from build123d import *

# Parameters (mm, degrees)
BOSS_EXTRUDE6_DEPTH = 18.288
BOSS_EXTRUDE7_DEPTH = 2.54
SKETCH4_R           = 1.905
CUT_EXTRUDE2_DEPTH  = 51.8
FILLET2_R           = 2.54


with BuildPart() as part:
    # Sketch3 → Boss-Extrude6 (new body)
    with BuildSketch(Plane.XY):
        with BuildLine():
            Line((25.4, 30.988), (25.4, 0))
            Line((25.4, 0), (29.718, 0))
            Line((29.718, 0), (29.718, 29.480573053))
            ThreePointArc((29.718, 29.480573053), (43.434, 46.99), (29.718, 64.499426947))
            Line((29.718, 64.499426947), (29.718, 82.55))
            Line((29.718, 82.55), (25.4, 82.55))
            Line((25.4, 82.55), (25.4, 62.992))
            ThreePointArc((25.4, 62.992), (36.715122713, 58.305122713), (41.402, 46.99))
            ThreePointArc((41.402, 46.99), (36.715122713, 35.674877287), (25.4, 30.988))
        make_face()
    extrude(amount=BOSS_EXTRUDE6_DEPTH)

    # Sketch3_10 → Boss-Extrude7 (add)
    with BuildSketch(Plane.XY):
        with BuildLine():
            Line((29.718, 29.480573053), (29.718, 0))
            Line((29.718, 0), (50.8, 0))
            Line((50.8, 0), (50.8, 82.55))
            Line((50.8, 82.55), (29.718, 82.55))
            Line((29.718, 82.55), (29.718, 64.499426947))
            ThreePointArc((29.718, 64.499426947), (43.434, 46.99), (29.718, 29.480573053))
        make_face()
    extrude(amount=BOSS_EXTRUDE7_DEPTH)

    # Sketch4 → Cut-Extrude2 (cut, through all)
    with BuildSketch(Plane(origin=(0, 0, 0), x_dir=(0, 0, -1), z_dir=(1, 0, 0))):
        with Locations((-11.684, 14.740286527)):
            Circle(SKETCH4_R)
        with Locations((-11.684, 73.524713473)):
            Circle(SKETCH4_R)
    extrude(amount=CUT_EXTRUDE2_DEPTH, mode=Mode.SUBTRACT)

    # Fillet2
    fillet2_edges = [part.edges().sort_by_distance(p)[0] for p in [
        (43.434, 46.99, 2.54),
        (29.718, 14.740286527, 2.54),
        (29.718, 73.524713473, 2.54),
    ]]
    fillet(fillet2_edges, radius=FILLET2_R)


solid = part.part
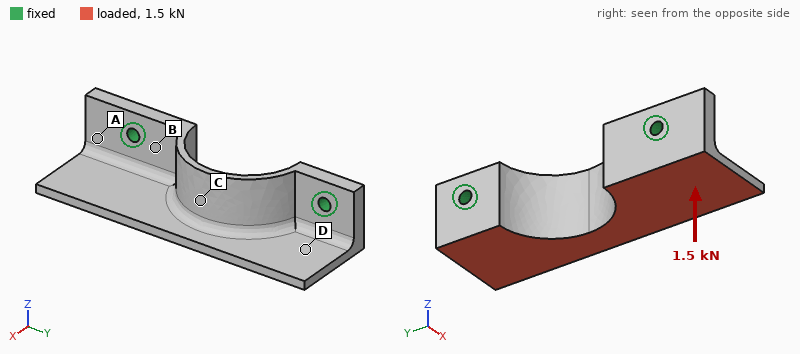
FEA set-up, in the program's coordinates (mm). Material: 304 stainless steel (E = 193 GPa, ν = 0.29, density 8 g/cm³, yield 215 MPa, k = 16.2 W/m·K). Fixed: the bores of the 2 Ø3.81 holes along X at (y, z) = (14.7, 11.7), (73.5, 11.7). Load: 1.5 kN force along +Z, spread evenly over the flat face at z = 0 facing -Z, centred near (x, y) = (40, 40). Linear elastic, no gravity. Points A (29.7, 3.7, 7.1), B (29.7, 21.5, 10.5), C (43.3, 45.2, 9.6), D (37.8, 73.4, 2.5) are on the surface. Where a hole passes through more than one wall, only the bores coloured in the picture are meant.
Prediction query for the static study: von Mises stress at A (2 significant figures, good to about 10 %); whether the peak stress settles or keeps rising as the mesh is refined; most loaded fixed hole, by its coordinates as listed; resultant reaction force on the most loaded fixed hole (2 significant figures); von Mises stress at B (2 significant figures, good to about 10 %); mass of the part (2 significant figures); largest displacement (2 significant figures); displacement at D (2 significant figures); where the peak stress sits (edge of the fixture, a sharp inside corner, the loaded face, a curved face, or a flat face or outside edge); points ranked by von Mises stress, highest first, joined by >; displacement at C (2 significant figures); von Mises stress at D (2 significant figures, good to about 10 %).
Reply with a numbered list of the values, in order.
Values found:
1. 60 MPa
2. keeps rising
3. (14.7, 11.7)
4. 820 N
5. 87 MPa
6. 74 g
7. 0.12 mm
8. 0.032 mm
9. edge of the fixture
10. B > A > D > C
11. 0.043 mm
12. 41 MPa
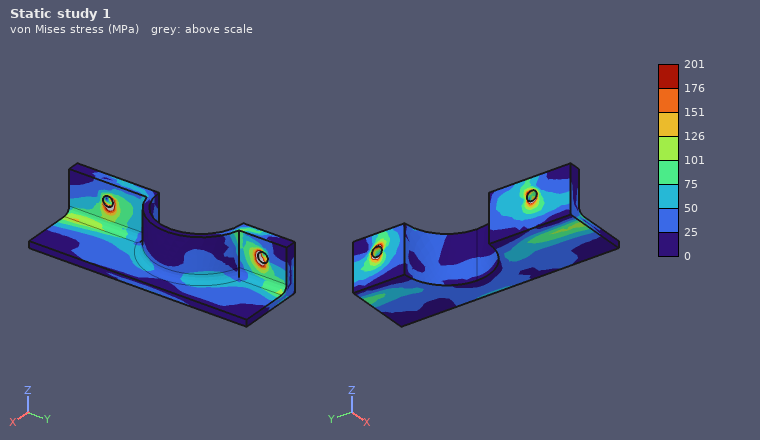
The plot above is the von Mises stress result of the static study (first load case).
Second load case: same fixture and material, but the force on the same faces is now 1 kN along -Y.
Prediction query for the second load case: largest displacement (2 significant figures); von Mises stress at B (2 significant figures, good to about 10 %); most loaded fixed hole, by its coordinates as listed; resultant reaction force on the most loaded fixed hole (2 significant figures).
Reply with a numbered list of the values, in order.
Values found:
1. 9.1 µm
2. 15 MPa
3. (14.7, 11.7)
4. 610 N
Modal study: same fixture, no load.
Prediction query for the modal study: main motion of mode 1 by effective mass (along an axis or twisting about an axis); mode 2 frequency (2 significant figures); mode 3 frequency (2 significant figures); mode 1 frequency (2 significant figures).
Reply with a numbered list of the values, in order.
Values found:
1. along Z
2. 4700 Hz
3. 6300 Hz
4. 3700 Hz
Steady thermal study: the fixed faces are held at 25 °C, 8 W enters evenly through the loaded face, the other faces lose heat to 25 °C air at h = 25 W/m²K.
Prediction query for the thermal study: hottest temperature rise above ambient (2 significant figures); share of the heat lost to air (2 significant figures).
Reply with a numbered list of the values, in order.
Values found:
1. 39 K
2. 34 %
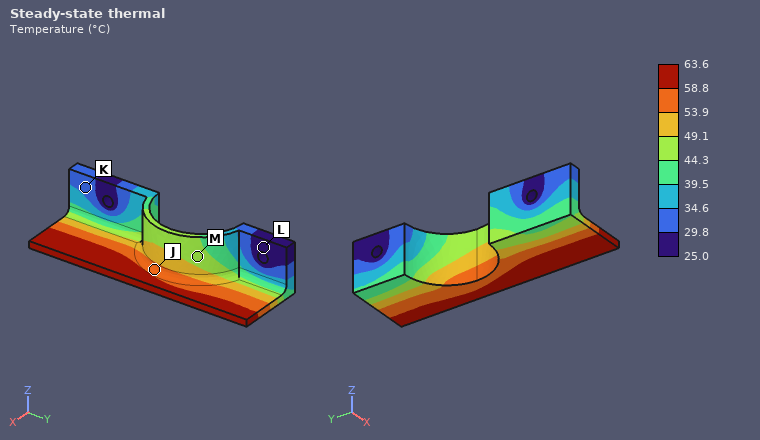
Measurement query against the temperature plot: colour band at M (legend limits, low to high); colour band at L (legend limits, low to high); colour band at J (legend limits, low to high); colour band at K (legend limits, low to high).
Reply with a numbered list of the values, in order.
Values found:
1. 44.3 to 49.1 °C
2. 25.0 to 29.8 °C
3. 53.9 to 58.8 °C
4. 29.8 to 34.6 °C
